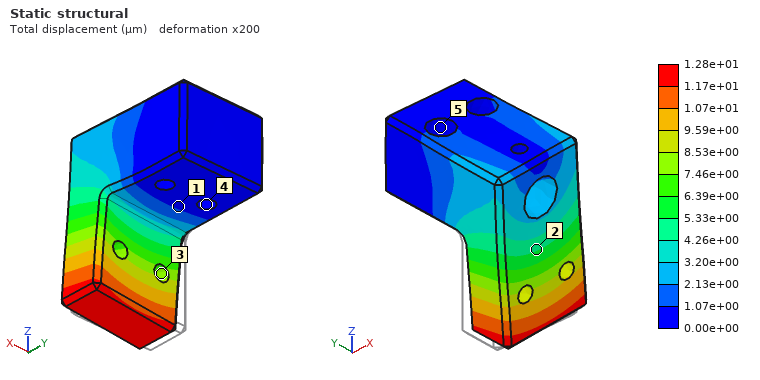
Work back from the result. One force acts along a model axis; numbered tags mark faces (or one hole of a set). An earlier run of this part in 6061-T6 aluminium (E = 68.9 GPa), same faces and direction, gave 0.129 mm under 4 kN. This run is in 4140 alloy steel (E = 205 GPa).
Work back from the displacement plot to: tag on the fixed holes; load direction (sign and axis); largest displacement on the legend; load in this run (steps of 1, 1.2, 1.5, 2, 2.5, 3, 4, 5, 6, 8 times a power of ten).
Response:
4
+X
1.28e+01 µm
1.2 kN
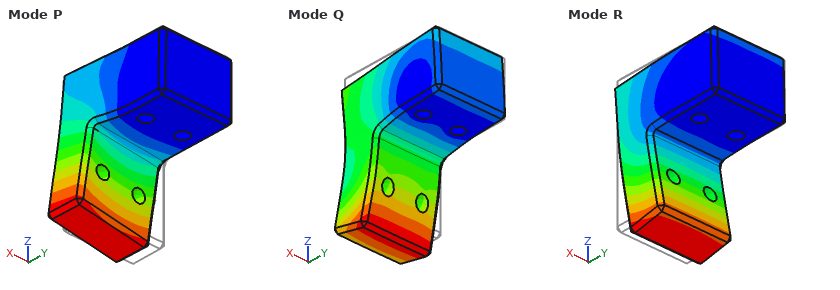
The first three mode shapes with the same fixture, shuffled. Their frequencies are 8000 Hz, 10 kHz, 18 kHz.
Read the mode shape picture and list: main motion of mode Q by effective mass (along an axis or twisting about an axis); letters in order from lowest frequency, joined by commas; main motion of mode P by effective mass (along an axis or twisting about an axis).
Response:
along Z
R, P, Q
along X
